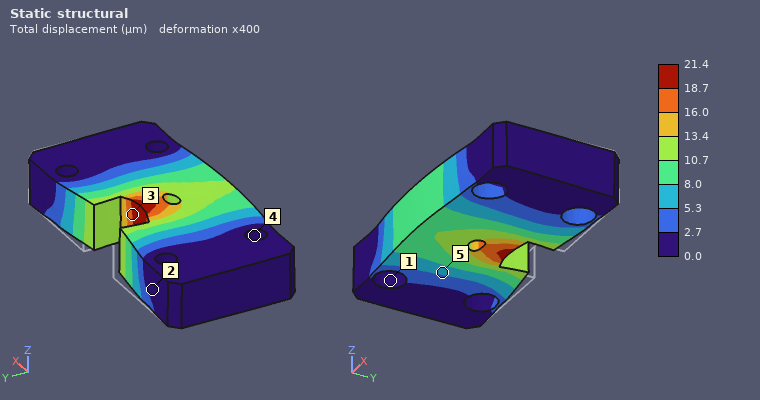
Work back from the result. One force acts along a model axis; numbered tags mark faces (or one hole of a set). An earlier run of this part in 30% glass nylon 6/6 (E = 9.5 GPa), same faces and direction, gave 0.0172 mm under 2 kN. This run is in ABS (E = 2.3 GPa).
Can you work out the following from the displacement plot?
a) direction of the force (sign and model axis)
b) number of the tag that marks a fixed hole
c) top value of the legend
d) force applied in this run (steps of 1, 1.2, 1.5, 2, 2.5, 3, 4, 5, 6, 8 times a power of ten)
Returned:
-Y
4
21.4 µm
600 N
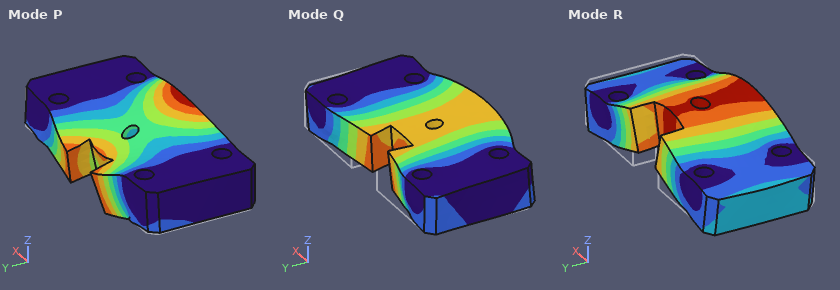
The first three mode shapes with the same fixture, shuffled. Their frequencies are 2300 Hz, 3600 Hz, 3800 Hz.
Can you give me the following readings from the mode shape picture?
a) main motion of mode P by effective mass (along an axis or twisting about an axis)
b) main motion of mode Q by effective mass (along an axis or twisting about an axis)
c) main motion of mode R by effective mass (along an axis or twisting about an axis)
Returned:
twisting about X
along Y
along Z
